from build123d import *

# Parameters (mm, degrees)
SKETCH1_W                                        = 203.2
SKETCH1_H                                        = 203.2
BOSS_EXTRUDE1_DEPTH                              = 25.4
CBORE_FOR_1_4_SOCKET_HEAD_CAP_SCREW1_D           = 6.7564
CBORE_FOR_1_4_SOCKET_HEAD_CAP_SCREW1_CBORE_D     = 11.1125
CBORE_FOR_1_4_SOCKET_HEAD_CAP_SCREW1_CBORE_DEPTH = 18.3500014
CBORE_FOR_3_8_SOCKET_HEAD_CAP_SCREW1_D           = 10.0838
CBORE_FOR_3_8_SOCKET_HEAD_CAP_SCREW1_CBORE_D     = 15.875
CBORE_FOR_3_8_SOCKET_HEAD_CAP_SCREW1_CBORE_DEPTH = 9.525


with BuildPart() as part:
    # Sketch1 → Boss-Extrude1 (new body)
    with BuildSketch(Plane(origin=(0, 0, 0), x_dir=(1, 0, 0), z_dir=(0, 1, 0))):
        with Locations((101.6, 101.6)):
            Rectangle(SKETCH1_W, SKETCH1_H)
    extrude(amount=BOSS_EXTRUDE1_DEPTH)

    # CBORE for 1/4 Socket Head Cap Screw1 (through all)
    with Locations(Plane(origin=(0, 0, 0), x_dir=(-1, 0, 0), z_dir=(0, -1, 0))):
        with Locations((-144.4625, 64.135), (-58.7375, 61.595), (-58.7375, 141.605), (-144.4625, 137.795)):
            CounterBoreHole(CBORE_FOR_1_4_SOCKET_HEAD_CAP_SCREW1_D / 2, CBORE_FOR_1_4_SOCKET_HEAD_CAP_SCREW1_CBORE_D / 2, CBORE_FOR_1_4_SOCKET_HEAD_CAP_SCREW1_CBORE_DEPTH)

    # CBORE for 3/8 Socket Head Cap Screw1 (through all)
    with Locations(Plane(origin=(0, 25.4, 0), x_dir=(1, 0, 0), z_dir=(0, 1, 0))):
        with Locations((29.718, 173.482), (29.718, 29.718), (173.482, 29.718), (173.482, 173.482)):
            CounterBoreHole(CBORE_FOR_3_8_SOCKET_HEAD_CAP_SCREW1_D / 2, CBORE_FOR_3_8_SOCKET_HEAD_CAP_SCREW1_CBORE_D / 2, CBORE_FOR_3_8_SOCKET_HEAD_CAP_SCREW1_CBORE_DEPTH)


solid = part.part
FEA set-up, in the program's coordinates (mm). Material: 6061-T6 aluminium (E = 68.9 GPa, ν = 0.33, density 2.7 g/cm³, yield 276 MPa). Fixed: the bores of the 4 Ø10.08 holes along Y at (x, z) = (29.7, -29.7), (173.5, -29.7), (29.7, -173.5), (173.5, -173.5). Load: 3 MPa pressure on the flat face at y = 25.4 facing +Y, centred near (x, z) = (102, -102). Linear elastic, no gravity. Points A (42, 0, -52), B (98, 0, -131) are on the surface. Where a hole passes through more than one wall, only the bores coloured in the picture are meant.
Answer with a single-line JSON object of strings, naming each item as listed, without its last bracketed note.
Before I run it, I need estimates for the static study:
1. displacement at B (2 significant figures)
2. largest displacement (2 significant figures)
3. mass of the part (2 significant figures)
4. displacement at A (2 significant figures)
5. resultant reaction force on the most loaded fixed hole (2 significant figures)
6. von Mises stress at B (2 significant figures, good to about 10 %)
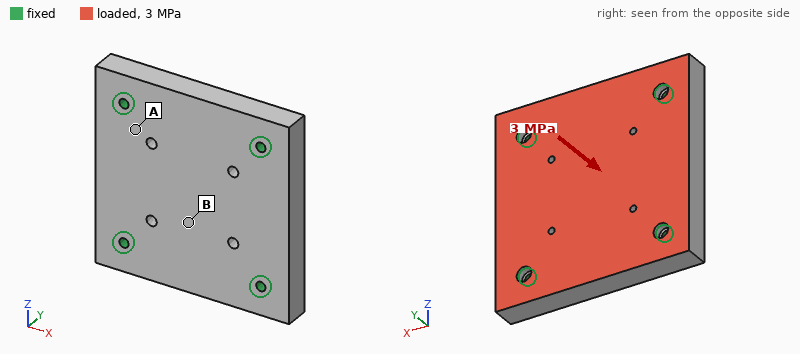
{"displacement at B": "0.14 mm", "largest displacement": "0.16 mm", "mass of the part": "2.8 kg", "displacement at A": "0.067 mm", "resultant reaction force on the most loaded fixed hole": "32 kN", "von Mises stress at B": "32 MPa"}
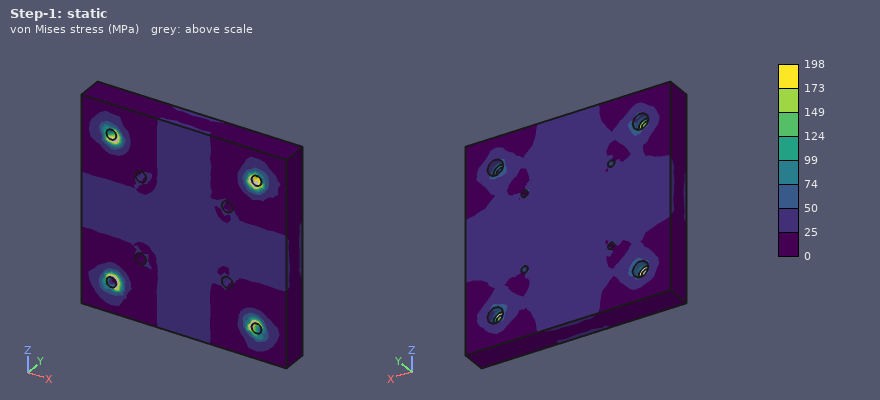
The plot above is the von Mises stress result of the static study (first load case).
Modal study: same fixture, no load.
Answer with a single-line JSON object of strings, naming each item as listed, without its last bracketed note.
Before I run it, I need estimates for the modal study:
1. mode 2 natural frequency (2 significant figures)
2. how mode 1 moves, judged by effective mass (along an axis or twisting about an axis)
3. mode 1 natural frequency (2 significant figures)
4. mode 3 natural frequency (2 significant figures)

{"mode 2 natural frequency": "4200 Hz", "how mode 1 moves, judged by effective mass": "along Y", "mode 1 natural frequency": "3100 Hz", "mode 3 natural frequency": "4500 Hz"}
